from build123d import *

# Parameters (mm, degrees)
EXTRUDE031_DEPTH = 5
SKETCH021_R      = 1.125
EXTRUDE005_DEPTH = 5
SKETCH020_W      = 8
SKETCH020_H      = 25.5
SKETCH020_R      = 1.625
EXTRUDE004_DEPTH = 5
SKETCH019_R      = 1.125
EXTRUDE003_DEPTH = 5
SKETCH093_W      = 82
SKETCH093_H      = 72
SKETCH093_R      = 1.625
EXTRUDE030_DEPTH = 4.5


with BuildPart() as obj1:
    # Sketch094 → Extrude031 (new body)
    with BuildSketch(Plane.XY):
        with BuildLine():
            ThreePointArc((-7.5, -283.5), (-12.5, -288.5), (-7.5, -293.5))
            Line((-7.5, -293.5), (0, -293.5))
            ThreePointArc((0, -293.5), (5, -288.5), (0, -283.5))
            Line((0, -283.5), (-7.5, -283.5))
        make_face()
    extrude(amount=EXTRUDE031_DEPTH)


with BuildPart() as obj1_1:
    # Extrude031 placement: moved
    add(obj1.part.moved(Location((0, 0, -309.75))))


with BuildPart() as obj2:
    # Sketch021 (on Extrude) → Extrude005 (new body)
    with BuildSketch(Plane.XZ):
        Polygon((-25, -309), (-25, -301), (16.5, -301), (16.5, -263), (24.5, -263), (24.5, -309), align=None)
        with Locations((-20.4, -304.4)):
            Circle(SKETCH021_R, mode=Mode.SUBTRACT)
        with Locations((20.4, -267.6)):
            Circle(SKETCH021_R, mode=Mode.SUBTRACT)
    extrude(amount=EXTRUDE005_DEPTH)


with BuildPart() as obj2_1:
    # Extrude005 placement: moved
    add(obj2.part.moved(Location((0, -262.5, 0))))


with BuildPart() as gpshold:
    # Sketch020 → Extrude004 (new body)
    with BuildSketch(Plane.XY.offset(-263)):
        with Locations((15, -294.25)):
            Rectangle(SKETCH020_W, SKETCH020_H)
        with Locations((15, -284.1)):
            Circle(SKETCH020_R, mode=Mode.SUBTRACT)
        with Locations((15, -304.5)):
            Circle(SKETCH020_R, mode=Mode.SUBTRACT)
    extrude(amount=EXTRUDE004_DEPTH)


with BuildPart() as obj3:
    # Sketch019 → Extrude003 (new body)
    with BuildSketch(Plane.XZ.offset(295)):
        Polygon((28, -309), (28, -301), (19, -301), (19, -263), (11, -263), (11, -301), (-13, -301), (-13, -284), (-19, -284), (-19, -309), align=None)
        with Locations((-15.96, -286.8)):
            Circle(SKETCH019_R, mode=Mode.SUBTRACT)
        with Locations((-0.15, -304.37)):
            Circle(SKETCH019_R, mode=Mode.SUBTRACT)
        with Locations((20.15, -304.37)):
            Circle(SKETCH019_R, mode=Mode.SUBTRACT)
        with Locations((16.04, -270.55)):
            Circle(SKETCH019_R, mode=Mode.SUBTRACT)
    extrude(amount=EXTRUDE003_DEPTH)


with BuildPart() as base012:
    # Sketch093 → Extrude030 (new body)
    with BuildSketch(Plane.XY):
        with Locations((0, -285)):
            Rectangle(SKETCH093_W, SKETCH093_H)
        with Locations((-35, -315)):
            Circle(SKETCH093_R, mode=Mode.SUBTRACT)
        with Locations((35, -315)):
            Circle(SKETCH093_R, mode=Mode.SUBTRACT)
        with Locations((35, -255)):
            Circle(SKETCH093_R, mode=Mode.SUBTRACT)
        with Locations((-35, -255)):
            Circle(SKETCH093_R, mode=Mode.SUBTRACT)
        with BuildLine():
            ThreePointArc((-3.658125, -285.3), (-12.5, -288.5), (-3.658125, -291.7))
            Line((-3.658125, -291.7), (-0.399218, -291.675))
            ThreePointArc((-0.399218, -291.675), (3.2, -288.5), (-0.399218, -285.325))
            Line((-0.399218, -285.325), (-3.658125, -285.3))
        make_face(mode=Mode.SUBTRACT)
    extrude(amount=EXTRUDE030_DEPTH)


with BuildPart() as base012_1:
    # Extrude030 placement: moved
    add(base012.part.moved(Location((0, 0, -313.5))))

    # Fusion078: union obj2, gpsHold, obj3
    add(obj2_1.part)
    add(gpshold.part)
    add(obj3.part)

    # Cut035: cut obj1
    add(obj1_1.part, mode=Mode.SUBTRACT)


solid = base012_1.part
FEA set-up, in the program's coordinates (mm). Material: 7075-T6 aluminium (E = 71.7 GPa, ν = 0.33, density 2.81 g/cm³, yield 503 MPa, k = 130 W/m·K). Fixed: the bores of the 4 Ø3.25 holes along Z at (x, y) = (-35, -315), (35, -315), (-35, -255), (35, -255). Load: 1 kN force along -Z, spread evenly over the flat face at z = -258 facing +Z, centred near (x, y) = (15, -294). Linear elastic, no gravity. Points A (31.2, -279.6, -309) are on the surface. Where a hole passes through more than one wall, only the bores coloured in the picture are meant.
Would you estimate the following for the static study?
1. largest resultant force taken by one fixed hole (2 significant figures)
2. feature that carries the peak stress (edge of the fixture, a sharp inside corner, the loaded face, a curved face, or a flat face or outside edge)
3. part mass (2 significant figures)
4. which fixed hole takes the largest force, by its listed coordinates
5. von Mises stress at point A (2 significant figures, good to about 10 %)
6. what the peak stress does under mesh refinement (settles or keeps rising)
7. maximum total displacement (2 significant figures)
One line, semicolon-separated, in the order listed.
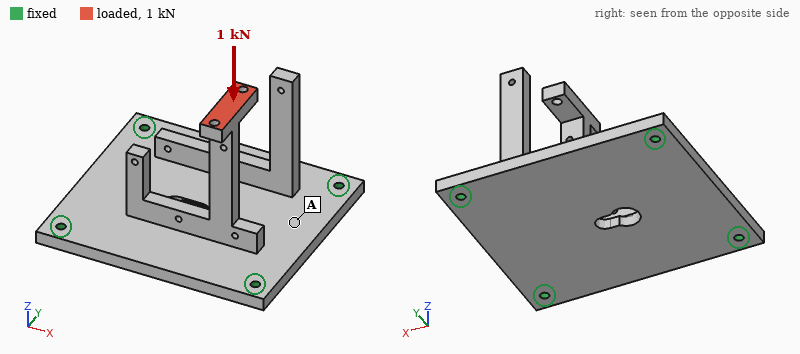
520 N; a sharp inside corner; 96 g; (35, -315); 18 MPa; keeps rising; 0.92 mm
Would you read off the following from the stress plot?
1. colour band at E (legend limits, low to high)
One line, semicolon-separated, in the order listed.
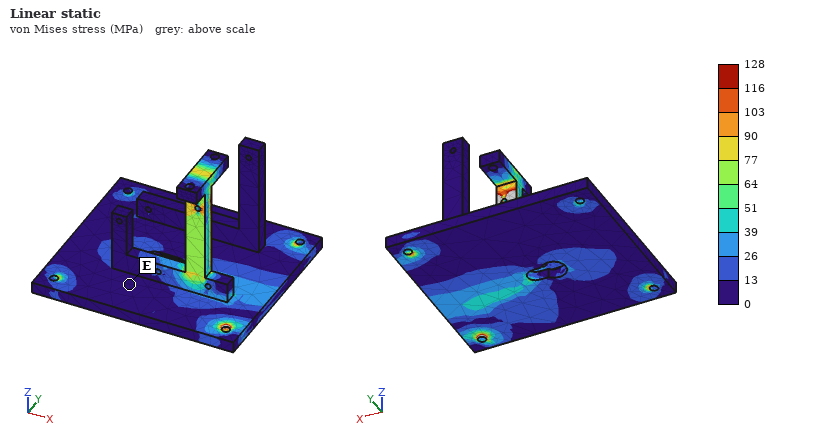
0 to 13 MPa
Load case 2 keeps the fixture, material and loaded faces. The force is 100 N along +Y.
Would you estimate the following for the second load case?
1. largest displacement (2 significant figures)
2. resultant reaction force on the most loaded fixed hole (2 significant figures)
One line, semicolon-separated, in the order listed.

0.79 mm; 88 N
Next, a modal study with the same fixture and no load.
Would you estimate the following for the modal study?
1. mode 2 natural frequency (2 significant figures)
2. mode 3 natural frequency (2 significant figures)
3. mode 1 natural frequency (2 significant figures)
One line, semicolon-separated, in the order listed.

1800 Hz; 1900 Hz; 1000 Hz
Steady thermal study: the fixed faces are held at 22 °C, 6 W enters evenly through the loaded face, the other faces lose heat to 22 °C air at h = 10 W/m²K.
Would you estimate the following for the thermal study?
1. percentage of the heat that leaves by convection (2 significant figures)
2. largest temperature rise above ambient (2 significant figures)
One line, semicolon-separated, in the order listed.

15 %; 57 K
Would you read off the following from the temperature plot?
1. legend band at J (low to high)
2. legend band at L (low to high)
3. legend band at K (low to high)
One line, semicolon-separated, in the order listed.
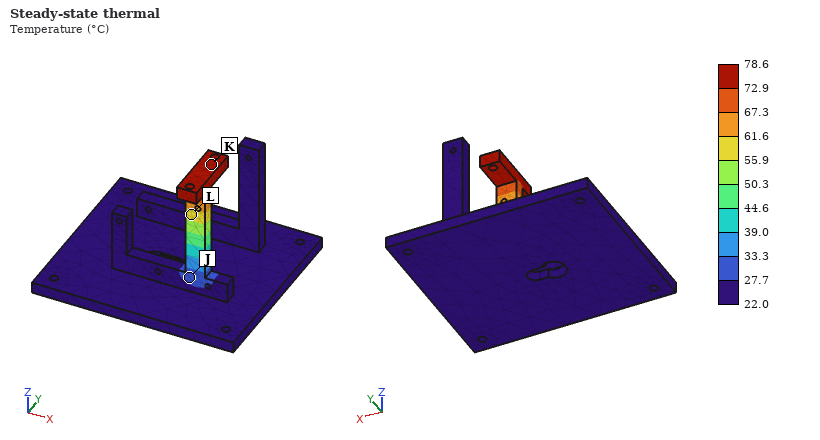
27.7 to 33.3 °C; 55.9 to 61.6 °C; 72.9 to 78.6 °C
